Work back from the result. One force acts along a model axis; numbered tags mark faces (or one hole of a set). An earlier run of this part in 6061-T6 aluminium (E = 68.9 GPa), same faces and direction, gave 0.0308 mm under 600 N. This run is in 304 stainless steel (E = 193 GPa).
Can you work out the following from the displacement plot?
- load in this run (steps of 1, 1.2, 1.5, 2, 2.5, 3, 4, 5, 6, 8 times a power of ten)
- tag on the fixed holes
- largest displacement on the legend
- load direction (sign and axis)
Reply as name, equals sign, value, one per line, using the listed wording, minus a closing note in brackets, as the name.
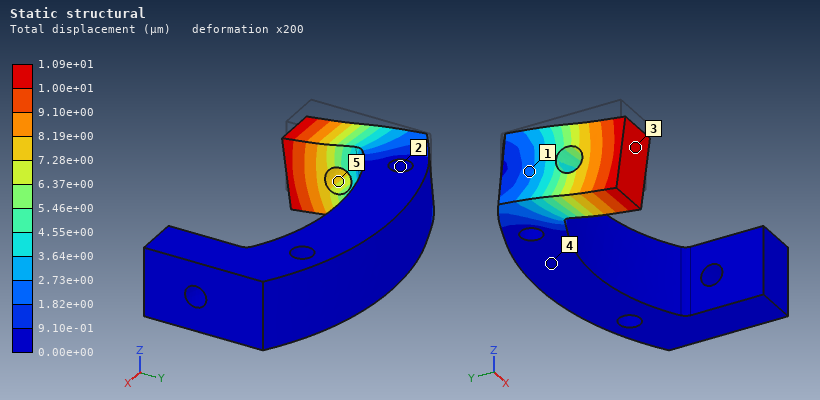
load in this run = 600 N
tag on the fixed holes = 2
largest displacement on the legend = 1.09e+01 µm
load direction = -Z
